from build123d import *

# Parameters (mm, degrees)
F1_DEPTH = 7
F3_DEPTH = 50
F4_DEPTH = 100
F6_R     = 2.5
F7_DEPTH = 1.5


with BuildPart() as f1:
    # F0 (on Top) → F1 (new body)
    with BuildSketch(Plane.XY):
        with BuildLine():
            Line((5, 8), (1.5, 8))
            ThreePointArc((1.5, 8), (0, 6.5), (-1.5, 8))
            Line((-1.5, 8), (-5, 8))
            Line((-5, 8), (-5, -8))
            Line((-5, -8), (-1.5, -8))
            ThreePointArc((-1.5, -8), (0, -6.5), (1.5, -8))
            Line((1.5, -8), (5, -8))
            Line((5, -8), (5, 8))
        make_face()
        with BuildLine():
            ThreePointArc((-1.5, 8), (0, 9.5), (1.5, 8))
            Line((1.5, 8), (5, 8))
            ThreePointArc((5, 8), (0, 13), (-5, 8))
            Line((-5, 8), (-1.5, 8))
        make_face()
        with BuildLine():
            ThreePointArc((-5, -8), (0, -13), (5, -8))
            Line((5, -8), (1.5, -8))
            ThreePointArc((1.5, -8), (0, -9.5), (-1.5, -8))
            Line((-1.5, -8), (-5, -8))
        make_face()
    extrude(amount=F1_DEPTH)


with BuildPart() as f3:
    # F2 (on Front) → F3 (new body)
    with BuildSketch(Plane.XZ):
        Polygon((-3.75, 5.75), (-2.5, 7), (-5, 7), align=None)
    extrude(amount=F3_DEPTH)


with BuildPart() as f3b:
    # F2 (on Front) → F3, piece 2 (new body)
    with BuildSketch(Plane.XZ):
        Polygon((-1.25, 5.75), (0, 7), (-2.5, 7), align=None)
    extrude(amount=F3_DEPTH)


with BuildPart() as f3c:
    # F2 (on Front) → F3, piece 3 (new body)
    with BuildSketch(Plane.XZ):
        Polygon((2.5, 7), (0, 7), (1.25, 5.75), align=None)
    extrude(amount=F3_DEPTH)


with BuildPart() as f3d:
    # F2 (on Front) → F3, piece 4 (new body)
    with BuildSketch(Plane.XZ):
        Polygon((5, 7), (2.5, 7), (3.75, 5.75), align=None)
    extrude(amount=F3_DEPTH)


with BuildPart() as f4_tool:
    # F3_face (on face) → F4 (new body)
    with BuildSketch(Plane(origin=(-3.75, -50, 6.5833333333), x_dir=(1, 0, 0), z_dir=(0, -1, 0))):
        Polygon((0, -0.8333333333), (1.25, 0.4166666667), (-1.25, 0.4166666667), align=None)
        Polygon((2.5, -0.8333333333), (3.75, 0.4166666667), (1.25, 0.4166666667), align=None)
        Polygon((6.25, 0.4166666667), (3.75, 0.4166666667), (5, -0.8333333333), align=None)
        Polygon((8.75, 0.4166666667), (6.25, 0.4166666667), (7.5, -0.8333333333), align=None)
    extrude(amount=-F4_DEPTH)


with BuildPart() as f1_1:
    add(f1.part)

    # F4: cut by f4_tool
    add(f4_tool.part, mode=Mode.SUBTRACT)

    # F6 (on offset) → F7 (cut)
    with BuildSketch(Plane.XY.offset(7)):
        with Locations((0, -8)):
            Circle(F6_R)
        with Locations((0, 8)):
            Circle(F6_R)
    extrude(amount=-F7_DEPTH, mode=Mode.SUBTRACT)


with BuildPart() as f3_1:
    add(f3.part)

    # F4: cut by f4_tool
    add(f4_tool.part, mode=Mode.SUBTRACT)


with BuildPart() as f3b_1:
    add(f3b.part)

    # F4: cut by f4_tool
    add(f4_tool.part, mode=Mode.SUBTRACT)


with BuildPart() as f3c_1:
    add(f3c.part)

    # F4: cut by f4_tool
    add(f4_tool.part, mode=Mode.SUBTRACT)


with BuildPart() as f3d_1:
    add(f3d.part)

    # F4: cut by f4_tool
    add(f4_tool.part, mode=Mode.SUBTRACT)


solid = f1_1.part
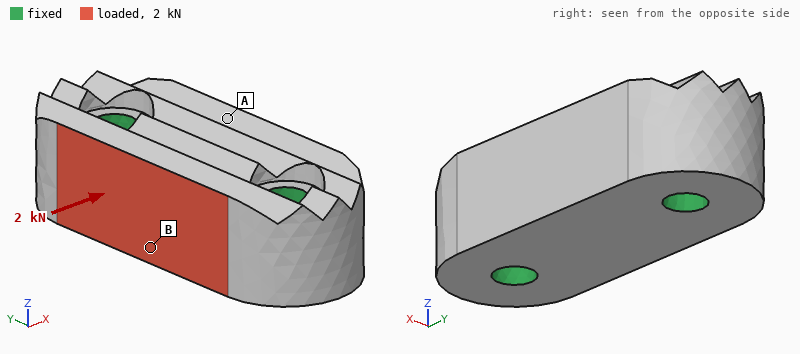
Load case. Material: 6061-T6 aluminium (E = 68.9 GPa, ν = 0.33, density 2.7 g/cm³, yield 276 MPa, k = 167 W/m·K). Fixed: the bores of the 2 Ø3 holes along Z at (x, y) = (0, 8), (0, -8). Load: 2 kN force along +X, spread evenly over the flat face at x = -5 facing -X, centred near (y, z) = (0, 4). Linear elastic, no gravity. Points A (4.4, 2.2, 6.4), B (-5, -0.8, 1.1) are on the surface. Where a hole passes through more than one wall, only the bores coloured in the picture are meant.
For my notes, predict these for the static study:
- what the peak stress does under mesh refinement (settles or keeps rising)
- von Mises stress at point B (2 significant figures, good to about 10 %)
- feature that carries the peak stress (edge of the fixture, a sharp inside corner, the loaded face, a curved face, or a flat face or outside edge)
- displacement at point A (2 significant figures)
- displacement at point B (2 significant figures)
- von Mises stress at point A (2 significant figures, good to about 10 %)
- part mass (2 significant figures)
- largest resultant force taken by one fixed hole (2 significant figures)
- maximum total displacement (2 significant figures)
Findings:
keeps rising
29 MPa
edge of the fixture
3.8 µm
4.0 µm
13 MPa
3.8 g
1.0 kN
12 µm
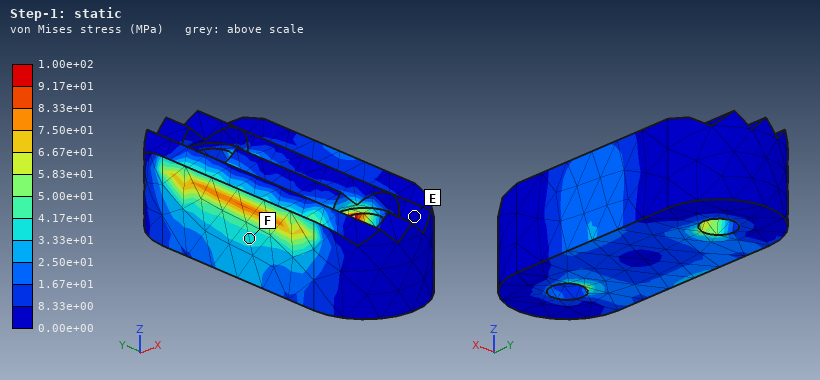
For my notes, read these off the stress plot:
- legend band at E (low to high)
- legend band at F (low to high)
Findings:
0.00e+00 to 8.33e+00 MPa
3.33e+01 to 4.17e+01 MPa
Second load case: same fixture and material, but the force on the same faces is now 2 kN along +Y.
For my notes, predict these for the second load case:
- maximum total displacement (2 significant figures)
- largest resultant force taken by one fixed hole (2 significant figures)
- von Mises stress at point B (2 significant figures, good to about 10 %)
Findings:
5.0 µm
1.1 kN
31 MPa
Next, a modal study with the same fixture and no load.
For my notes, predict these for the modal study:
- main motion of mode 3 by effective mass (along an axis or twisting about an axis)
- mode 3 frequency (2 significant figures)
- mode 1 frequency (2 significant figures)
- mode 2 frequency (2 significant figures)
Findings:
along X
77 kHz
70 kHz
70 kHz
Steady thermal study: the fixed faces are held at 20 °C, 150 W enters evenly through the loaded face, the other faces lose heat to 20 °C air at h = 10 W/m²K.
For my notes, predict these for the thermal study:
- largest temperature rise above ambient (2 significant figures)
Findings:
75 K
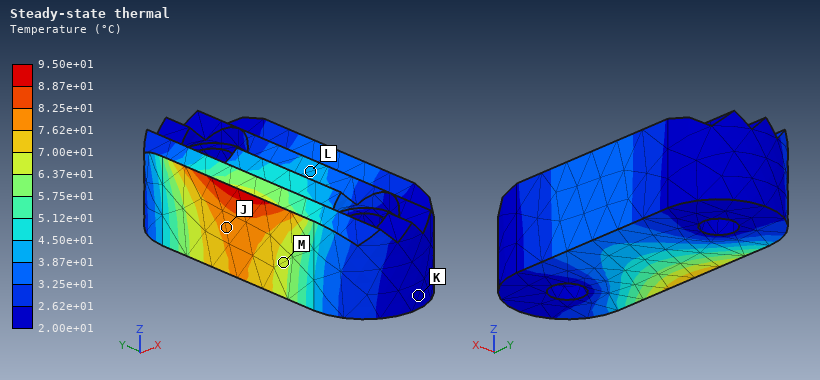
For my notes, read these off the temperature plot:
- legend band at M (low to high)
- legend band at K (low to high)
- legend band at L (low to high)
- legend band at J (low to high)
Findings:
6.37e+01 to 7.00e+01 °C
2.00e+01 to 2.62e+01 °C
3.87e+01 to 4.50e+01 °C
7.62e+01 to 8.25e+01 °C
